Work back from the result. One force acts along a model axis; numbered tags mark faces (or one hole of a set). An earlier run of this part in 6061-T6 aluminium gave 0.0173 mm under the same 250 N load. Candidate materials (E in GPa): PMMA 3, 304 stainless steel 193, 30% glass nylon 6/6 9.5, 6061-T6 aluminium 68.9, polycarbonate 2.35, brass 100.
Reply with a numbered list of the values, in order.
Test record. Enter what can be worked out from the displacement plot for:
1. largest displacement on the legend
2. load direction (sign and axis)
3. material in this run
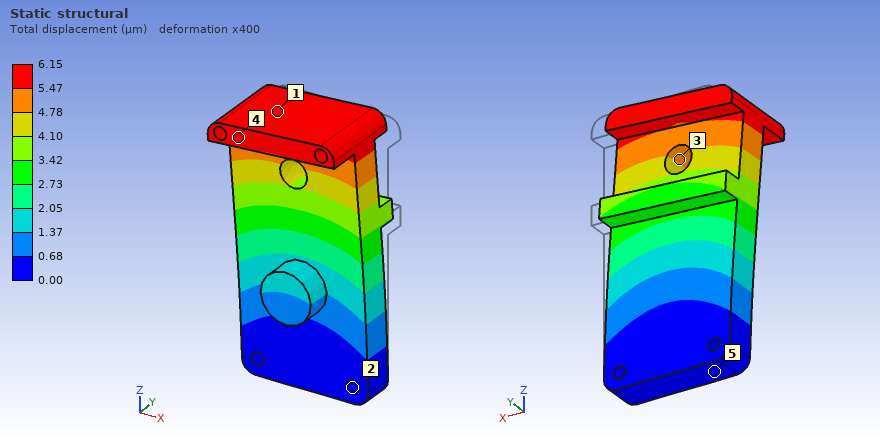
1. 6.15 µm
2. -X
3. 304 stainless steel
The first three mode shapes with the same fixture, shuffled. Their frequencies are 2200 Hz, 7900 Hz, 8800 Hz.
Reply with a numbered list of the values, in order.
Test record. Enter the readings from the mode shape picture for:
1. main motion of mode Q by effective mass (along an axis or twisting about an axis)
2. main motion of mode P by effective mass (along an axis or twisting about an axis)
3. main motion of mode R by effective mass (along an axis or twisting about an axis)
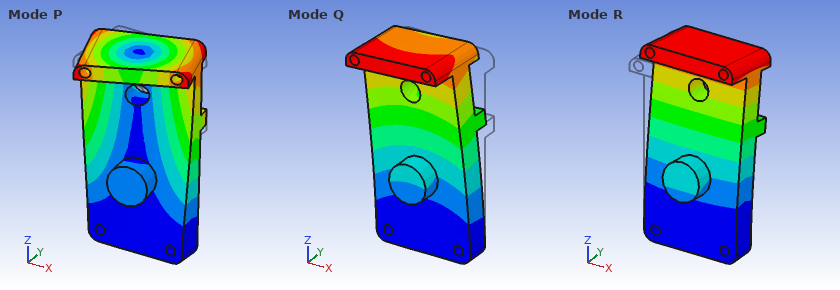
1. along X
2. twisting about Z
3. along Y
